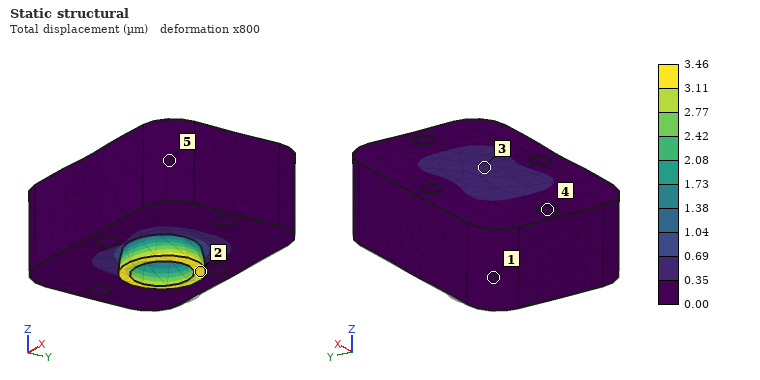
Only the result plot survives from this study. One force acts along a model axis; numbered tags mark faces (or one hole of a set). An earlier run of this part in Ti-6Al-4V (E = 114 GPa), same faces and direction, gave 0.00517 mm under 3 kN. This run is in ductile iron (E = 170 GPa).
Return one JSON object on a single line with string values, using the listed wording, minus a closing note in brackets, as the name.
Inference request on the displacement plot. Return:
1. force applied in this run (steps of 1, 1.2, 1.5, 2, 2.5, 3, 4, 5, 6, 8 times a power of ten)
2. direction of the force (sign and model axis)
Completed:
{"force applied in this run": "3 kN", "direction of the force": "+Z"}
